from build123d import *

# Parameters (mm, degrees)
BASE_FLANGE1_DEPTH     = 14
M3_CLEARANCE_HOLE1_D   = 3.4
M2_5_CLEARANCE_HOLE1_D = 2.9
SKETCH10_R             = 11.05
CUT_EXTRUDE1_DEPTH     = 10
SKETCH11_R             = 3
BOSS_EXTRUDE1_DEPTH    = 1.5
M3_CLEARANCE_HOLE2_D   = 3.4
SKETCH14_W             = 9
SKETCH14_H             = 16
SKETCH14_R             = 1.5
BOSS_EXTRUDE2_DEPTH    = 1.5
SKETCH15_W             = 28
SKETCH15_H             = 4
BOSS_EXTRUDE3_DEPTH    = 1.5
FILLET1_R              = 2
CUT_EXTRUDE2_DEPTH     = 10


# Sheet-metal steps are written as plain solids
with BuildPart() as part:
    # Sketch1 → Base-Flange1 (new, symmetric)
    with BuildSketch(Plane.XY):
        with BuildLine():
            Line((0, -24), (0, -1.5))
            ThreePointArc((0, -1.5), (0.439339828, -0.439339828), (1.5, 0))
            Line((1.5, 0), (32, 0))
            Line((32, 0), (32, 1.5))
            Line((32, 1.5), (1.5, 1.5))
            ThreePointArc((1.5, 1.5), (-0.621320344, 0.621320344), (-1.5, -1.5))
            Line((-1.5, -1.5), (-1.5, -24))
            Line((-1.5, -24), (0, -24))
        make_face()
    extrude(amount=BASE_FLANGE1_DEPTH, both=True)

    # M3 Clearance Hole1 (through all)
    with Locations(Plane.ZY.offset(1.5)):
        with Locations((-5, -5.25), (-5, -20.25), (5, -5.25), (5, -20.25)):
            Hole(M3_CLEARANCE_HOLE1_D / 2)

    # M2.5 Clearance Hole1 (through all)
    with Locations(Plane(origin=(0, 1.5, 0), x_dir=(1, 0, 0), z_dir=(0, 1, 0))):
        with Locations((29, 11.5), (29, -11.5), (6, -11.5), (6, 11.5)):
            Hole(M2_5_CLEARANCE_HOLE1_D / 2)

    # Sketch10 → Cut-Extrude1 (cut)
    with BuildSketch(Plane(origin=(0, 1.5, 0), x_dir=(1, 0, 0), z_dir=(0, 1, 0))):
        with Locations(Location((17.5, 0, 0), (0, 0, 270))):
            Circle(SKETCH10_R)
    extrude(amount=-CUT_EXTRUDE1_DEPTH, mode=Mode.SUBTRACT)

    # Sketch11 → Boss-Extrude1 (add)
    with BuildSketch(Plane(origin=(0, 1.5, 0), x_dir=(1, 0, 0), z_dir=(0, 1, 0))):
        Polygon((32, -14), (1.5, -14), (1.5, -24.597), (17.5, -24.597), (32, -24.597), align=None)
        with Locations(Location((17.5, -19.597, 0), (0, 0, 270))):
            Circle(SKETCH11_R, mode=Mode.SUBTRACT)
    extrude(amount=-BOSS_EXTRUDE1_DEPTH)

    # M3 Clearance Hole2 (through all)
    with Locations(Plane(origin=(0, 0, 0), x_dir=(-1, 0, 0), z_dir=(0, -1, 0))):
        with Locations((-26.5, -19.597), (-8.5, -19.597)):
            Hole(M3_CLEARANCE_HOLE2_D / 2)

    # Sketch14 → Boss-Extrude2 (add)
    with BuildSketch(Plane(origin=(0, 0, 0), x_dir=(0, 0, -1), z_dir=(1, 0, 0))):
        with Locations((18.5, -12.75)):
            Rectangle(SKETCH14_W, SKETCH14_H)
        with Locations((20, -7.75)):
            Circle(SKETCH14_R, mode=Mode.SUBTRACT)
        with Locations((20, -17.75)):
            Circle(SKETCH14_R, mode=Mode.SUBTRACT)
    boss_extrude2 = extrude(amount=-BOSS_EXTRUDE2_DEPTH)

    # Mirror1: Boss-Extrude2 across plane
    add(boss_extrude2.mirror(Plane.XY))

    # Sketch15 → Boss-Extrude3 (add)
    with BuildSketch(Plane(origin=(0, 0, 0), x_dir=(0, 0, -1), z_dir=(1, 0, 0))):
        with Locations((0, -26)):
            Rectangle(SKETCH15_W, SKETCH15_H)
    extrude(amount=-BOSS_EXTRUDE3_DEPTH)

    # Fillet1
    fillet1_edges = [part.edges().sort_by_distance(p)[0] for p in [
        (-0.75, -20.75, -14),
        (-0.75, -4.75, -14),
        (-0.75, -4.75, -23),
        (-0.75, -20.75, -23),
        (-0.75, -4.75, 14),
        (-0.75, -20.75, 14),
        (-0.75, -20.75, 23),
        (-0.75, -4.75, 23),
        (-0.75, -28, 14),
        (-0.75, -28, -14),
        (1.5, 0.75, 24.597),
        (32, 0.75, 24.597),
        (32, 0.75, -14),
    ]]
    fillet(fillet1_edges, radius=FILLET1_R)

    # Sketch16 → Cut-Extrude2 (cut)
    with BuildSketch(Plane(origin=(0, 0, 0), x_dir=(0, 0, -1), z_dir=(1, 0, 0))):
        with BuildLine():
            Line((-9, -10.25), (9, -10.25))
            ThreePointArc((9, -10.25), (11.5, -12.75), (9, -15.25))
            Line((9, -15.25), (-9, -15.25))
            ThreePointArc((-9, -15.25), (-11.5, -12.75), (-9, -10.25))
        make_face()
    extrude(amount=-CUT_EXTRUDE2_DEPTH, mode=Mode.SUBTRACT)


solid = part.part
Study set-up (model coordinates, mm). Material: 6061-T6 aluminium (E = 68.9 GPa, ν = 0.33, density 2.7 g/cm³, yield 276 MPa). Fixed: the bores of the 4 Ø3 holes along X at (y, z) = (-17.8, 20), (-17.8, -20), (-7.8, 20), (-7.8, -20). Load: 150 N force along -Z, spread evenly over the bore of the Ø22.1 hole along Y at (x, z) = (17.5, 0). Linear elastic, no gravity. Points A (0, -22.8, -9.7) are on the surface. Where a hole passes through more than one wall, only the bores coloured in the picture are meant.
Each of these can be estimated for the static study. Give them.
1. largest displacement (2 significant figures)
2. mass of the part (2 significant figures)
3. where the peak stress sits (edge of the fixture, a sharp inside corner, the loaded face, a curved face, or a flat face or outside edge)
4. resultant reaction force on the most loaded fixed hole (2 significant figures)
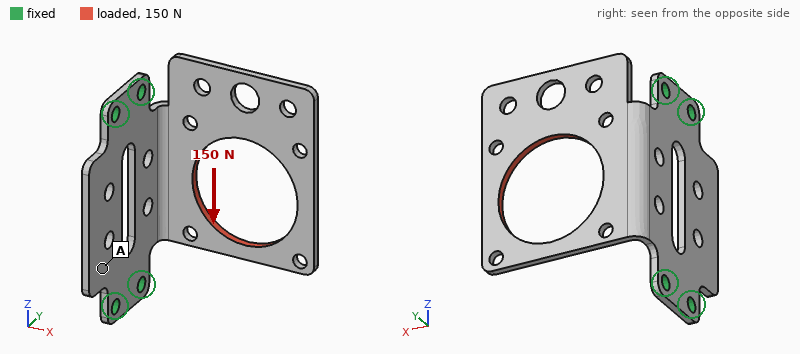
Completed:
0.53 mm
6.8 g
a curved face
130 N
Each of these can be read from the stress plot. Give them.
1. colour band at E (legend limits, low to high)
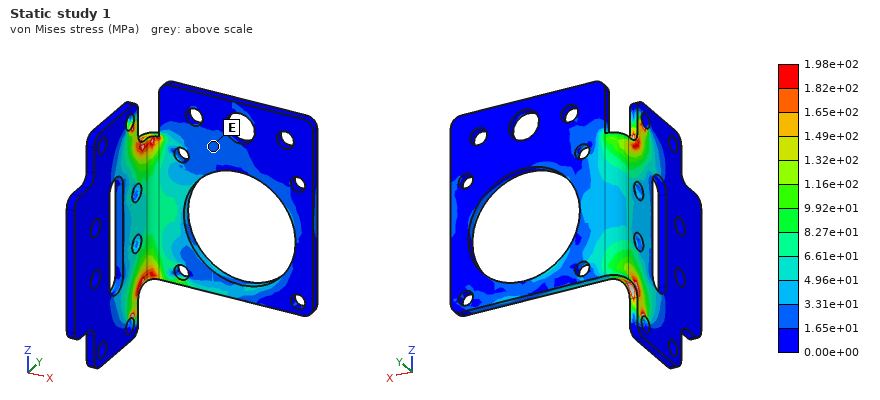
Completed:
1.65e+01 to 3.31e+01 MPa
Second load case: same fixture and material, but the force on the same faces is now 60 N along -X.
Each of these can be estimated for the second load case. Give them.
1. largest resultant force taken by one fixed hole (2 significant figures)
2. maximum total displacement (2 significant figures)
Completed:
46 N
0.34 mm
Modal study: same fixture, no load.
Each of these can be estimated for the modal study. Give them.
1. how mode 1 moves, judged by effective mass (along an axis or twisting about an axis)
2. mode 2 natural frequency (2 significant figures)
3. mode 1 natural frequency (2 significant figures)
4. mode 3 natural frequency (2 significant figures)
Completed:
along Y
1600 Hz
630 Hz
2100 Hz
